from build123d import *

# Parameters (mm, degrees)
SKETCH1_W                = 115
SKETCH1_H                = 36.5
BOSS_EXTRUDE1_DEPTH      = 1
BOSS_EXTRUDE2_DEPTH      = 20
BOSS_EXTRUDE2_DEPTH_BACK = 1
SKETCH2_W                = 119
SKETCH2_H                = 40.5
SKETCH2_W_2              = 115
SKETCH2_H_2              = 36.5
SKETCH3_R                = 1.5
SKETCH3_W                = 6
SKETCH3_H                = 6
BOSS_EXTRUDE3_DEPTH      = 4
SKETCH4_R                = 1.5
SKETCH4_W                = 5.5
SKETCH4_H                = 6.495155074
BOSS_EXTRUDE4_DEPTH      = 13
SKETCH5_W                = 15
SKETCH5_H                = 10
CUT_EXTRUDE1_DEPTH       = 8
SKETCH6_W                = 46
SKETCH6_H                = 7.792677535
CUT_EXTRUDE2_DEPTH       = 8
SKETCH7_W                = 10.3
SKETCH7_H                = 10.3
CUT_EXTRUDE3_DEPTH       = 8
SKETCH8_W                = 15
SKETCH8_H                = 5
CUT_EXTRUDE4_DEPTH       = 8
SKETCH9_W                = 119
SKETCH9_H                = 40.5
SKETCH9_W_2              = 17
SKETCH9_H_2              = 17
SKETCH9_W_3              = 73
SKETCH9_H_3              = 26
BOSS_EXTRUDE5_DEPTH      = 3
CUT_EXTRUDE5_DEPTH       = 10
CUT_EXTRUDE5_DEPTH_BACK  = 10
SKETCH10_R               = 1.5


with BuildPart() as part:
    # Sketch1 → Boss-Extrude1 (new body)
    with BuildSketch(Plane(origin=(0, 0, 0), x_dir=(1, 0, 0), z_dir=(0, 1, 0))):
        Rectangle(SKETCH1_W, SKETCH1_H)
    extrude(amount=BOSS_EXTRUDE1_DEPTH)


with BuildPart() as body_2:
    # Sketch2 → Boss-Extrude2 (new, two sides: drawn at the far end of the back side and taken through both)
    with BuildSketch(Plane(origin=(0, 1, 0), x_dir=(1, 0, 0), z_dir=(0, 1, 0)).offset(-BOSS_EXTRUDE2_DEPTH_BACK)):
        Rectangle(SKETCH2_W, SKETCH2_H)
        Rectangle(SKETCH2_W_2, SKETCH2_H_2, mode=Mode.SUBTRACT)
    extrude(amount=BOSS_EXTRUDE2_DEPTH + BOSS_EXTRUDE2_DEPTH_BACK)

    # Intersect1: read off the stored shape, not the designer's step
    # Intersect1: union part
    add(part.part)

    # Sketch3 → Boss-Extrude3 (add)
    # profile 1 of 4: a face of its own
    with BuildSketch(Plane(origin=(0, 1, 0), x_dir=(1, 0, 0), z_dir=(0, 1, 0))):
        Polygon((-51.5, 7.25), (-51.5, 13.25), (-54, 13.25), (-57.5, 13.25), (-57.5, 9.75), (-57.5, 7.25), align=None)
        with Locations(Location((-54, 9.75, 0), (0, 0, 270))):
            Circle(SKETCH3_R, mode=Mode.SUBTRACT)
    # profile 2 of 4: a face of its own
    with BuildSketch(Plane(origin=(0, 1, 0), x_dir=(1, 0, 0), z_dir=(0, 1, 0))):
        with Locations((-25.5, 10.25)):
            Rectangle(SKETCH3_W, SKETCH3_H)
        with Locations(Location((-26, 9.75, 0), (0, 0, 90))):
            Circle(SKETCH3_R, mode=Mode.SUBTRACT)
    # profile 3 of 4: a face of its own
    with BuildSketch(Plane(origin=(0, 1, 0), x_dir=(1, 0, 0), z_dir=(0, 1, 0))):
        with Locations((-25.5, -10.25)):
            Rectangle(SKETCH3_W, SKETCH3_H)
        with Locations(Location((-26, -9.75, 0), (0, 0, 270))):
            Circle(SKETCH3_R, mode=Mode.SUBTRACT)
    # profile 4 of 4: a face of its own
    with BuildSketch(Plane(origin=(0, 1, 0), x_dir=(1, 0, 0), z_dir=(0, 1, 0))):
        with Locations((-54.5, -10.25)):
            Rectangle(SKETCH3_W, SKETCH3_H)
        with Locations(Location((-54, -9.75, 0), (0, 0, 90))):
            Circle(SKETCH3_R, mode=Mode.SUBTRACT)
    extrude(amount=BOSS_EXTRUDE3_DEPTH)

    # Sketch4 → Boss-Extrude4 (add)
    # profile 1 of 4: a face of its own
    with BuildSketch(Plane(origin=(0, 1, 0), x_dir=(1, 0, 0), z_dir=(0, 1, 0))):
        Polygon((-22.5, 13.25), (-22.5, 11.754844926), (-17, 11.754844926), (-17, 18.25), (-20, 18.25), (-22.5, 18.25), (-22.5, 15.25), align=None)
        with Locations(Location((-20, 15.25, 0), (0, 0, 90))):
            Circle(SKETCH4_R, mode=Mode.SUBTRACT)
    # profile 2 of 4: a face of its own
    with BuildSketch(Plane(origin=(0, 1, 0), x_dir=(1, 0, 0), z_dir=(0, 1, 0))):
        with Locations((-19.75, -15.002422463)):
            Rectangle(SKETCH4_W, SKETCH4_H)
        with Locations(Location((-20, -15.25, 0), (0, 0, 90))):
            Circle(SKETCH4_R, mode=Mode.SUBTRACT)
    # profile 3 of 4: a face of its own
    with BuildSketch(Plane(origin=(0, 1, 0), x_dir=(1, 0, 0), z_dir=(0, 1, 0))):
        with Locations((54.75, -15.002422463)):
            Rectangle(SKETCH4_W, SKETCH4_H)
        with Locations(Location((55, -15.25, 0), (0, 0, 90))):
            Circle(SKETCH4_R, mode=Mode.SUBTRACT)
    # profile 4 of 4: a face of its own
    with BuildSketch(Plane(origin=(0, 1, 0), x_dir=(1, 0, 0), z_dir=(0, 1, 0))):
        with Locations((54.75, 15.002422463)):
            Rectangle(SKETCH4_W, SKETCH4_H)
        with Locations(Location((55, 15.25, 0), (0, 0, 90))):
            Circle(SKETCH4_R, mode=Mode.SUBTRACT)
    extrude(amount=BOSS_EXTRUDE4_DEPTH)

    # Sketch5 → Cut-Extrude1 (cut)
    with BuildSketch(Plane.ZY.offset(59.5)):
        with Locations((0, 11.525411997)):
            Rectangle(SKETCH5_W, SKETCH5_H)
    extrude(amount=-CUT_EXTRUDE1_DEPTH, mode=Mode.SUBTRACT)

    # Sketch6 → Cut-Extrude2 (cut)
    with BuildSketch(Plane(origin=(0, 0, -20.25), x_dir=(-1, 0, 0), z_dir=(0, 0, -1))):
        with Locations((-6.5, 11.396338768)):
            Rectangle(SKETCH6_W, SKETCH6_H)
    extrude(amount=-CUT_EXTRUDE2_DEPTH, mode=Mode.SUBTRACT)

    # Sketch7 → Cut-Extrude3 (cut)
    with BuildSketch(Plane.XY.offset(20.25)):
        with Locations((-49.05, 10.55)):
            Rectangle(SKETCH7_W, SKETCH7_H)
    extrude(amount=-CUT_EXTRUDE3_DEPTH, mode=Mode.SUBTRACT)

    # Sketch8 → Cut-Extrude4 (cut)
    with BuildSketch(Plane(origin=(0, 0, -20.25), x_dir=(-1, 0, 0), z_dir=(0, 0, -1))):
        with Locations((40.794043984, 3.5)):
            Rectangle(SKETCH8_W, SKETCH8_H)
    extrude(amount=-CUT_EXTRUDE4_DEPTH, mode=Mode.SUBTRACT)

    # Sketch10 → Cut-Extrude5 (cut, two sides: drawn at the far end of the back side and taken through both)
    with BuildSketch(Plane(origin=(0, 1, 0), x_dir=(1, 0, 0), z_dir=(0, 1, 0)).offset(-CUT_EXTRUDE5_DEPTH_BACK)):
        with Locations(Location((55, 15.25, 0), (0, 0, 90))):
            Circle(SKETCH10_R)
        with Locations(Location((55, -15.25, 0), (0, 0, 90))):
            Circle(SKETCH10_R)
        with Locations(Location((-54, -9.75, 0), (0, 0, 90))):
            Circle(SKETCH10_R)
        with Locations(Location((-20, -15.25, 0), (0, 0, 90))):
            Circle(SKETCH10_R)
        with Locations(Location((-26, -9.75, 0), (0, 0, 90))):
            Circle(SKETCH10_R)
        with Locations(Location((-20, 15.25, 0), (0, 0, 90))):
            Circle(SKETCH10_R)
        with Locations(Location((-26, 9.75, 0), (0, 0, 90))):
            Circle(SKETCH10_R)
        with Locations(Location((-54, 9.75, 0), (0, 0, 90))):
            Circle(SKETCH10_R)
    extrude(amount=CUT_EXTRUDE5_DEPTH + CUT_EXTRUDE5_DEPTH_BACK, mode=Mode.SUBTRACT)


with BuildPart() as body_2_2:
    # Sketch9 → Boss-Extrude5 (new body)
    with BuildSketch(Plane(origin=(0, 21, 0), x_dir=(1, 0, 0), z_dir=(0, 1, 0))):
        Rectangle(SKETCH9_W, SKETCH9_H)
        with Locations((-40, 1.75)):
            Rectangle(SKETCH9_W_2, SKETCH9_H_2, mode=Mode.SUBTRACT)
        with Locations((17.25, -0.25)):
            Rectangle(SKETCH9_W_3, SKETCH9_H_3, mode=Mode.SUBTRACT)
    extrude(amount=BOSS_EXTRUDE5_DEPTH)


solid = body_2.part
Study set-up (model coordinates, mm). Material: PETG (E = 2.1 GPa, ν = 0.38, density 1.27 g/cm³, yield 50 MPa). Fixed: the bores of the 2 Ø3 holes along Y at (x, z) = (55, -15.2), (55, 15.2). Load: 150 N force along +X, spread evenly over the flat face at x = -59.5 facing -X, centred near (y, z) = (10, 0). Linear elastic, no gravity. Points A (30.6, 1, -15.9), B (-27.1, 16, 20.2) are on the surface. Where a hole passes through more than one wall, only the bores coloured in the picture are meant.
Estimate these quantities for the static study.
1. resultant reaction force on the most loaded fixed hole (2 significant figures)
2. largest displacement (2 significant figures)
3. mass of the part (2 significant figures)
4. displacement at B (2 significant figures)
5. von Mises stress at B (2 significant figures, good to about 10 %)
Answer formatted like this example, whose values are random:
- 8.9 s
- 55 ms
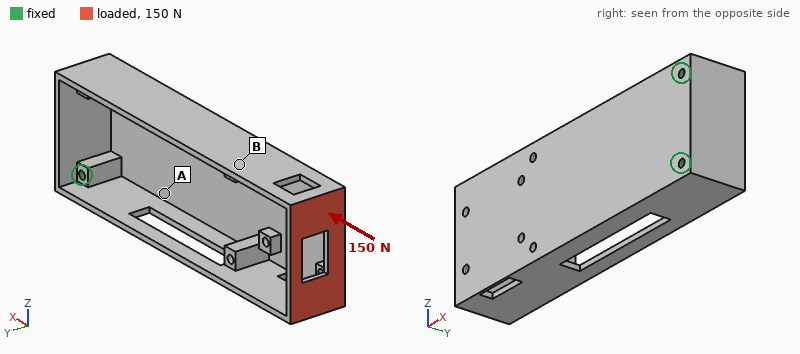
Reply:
- 76 N
- 1.3 mm
- 23 g
- 0.30 mm
- 2.5 MPa
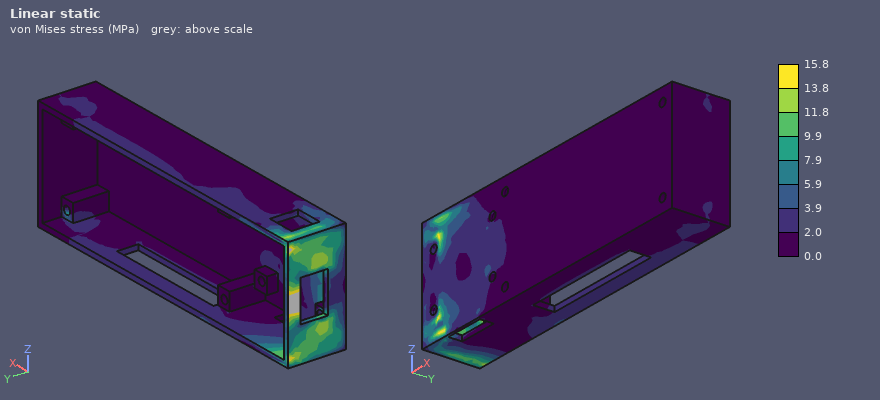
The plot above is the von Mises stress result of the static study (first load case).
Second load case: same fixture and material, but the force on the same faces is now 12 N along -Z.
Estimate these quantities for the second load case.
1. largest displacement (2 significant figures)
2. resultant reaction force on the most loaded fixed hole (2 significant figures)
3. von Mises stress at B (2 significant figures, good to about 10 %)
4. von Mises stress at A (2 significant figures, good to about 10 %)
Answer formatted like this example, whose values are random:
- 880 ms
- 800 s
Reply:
- 1.3 mm
- 42 N
- 0.97 MPa
- 2.2 MPa
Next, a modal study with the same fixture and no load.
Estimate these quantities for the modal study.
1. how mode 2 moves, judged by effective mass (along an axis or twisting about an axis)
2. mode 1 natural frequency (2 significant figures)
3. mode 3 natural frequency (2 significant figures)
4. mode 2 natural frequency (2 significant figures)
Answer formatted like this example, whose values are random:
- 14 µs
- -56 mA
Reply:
- along Y
- 190 Hz
- 440 Hz
- 230 Hz
